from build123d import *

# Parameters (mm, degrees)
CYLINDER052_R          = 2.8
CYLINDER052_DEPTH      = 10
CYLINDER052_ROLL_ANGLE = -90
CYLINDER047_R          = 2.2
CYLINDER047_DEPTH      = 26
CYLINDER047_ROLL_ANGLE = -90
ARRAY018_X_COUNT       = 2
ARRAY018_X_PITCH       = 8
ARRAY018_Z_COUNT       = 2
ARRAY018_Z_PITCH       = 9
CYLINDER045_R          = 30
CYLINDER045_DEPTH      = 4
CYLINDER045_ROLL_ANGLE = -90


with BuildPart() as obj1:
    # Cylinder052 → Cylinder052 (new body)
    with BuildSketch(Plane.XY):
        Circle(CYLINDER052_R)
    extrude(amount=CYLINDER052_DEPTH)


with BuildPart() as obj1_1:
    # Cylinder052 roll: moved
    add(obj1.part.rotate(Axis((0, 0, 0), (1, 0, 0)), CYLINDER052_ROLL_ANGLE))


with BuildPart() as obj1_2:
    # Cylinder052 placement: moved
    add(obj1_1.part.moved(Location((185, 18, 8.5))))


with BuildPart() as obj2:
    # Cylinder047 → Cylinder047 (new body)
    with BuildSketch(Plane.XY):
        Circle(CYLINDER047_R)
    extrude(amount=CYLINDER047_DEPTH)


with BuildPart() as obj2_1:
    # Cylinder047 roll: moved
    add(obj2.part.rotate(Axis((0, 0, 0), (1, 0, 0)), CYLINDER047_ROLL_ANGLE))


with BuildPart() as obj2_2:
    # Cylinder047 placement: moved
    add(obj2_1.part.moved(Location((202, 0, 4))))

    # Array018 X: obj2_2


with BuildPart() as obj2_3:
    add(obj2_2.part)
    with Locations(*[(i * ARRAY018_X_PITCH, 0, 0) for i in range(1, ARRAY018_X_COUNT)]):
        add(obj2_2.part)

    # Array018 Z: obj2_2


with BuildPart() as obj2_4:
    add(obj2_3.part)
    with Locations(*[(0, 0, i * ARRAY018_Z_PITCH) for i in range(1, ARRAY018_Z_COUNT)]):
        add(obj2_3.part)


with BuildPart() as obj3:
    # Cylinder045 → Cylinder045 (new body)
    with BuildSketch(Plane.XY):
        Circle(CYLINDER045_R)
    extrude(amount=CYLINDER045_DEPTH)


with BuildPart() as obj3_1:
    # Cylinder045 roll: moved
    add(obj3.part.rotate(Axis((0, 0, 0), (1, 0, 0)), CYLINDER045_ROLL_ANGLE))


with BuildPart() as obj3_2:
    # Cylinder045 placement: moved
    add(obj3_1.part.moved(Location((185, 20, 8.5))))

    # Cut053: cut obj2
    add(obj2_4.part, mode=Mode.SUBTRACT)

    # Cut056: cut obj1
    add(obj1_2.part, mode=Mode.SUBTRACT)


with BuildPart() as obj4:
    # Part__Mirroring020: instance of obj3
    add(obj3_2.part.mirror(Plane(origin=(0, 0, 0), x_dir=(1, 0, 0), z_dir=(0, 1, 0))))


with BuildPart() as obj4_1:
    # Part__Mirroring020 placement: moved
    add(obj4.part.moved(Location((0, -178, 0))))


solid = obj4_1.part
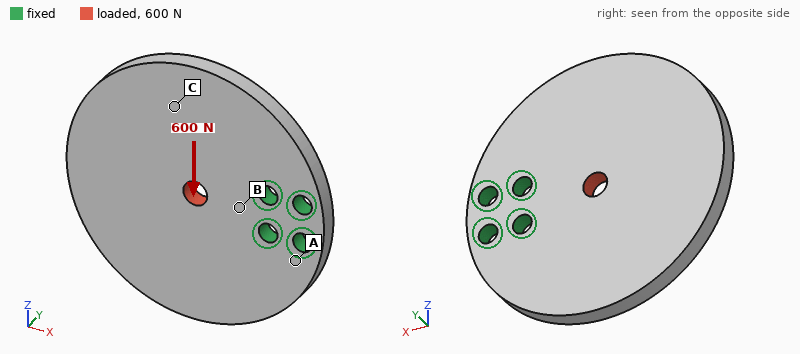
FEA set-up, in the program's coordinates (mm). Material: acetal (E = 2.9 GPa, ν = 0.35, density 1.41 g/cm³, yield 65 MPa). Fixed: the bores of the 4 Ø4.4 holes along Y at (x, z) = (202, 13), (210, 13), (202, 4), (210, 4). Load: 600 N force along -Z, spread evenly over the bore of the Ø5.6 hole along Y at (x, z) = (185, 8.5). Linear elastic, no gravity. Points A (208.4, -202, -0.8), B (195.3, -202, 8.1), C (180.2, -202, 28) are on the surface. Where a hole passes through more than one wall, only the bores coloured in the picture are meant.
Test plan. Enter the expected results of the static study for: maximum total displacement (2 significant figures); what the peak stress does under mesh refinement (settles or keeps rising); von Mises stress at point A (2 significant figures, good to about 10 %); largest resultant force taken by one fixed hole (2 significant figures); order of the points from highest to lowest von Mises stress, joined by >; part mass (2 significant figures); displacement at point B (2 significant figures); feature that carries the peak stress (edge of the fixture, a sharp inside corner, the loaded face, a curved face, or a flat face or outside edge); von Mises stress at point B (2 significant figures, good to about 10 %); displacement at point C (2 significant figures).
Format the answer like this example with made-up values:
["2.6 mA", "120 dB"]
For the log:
["0.30 mm", "keeps rising", "8.8 MPa", "610 N", "B > A > C", "15 g", "0.049 mm", "edge of the fixture", "15 MPa", "0.20 mm"]
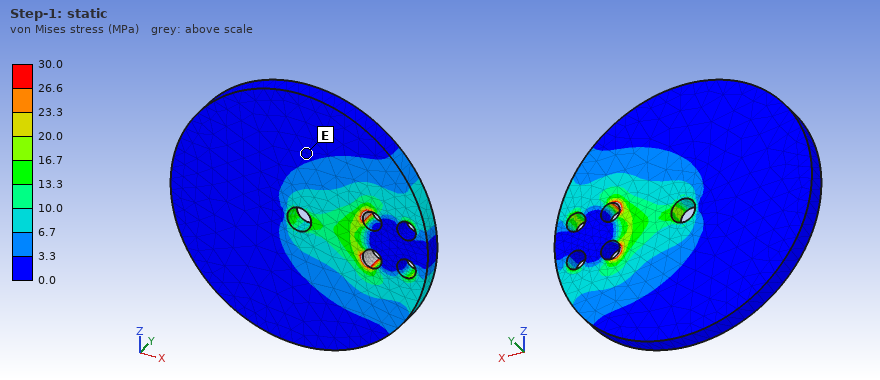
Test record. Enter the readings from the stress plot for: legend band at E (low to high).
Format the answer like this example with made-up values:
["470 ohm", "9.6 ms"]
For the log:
["0.0 to 3.3 MPa"]
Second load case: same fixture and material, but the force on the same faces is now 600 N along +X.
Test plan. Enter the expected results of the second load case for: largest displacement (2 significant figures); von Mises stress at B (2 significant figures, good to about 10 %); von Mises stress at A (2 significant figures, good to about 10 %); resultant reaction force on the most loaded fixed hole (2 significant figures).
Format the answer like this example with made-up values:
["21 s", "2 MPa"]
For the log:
["52 µm", "7.1 MPa", "2.3 MPa", "270 N"]
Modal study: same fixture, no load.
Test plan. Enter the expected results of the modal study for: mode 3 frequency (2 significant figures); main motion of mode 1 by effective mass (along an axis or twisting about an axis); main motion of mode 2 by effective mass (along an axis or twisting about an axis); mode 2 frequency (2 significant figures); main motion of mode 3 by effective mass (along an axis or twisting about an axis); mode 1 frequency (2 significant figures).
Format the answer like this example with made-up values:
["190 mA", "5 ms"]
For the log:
["1600 Hz", "along Y", "twisting about X", "810 Hz", "along Y", "470 Hz"]
